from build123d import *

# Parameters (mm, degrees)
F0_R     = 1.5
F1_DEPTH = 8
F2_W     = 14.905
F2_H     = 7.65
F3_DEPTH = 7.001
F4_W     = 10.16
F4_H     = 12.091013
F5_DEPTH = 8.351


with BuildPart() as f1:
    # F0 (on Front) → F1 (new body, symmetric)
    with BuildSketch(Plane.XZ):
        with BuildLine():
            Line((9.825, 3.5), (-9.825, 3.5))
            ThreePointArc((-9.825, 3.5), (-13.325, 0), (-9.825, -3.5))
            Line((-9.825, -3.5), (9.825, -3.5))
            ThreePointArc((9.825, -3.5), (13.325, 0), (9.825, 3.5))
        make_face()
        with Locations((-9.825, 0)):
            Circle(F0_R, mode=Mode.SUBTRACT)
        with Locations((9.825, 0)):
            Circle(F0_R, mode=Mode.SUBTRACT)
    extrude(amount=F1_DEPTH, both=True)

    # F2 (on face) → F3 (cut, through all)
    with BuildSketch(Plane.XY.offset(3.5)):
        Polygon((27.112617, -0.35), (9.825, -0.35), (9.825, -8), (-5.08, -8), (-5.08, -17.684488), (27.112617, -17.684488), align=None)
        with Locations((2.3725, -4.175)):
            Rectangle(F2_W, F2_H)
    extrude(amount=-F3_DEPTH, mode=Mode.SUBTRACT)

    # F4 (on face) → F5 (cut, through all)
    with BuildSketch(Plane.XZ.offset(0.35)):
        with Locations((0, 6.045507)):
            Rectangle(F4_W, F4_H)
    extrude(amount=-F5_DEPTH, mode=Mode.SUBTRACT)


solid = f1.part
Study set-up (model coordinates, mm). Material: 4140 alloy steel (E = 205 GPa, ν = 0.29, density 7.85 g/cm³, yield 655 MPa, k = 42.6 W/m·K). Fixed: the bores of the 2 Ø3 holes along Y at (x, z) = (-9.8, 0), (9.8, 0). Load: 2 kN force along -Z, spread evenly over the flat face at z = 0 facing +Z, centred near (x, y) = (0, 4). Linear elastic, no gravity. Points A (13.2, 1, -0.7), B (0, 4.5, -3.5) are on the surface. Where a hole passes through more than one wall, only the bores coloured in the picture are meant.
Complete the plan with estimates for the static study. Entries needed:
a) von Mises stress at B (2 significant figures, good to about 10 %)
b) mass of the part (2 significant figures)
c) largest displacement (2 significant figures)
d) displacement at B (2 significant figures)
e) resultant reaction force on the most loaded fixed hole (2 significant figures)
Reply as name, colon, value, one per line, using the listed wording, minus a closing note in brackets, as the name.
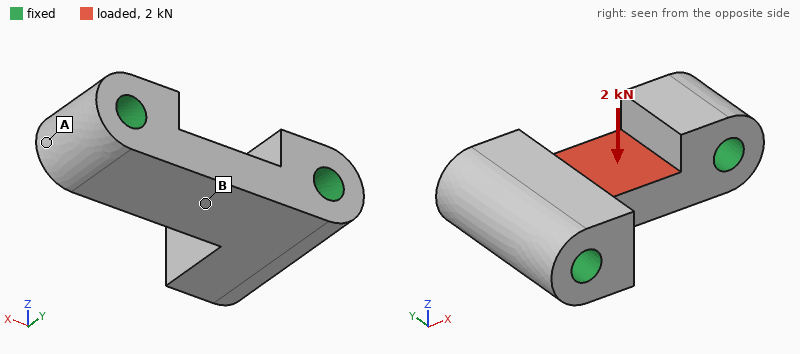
von Mises stress at B: 110 MPa
mass of the part: 11 g
largest displacement: 6.4 µm
displacement at B: 5.5 µm
resultant reaction force on the most loaded fixed hole: 1.1 kN
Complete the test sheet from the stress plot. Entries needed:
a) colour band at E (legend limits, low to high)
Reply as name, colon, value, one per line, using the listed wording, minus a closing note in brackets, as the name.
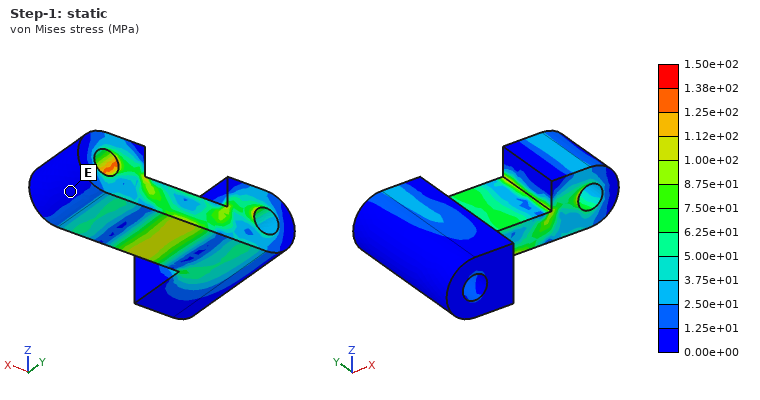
colour band at E: 0.00e+00 to 1.25e+01 MPa
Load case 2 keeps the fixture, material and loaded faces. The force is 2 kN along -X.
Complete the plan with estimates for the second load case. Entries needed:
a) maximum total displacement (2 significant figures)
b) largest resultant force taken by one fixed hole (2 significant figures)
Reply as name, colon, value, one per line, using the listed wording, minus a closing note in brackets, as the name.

maximum total displacement: 1.7 µm
largest resultant force taken by one fixed hole: 1.0 kN
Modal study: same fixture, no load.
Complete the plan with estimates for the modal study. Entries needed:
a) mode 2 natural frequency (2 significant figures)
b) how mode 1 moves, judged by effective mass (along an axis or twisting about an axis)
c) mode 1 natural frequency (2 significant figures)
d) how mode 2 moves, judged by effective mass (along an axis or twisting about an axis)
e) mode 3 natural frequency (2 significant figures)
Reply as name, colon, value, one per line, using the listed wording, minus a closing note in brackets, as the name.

mode 2 natural frequency: 82 kHz
how mode 1 moves, judged by effective mass: along Z
mode 1 natural frequency: 63 kHz
how mode 2 moves, judged by effective mass: along Y
mode 3 natural frequency: 91 kHz
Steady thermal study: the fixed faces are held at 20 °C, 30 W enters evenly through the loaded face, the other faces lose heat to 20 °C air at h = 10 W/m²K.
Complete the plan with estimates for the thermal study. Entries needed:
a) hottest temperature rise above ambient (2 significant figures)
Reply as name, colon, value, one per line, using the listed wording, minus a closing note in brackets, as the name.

hottest temperature rise above ambient: 71 K
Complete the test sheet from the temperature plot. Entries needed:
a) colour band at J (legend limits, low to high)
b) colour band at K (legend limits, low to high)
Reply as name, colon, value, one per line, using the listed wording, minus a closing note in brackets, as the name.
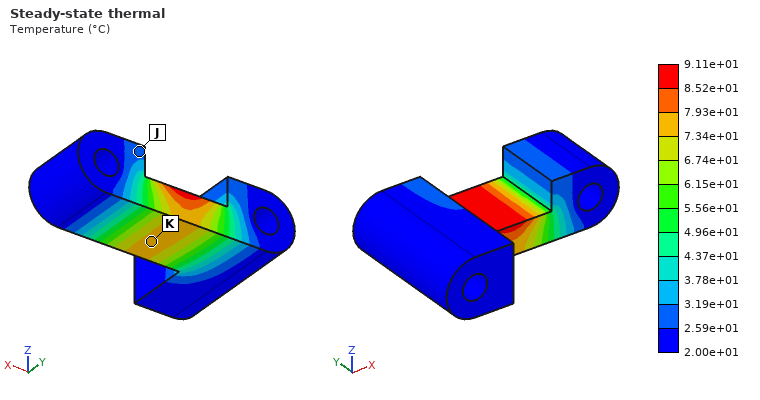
colour band at J: 2.59e+01 to 3.19e+01 °C
colour band at K: 7.34e+01 to 7.93e+01 °C
